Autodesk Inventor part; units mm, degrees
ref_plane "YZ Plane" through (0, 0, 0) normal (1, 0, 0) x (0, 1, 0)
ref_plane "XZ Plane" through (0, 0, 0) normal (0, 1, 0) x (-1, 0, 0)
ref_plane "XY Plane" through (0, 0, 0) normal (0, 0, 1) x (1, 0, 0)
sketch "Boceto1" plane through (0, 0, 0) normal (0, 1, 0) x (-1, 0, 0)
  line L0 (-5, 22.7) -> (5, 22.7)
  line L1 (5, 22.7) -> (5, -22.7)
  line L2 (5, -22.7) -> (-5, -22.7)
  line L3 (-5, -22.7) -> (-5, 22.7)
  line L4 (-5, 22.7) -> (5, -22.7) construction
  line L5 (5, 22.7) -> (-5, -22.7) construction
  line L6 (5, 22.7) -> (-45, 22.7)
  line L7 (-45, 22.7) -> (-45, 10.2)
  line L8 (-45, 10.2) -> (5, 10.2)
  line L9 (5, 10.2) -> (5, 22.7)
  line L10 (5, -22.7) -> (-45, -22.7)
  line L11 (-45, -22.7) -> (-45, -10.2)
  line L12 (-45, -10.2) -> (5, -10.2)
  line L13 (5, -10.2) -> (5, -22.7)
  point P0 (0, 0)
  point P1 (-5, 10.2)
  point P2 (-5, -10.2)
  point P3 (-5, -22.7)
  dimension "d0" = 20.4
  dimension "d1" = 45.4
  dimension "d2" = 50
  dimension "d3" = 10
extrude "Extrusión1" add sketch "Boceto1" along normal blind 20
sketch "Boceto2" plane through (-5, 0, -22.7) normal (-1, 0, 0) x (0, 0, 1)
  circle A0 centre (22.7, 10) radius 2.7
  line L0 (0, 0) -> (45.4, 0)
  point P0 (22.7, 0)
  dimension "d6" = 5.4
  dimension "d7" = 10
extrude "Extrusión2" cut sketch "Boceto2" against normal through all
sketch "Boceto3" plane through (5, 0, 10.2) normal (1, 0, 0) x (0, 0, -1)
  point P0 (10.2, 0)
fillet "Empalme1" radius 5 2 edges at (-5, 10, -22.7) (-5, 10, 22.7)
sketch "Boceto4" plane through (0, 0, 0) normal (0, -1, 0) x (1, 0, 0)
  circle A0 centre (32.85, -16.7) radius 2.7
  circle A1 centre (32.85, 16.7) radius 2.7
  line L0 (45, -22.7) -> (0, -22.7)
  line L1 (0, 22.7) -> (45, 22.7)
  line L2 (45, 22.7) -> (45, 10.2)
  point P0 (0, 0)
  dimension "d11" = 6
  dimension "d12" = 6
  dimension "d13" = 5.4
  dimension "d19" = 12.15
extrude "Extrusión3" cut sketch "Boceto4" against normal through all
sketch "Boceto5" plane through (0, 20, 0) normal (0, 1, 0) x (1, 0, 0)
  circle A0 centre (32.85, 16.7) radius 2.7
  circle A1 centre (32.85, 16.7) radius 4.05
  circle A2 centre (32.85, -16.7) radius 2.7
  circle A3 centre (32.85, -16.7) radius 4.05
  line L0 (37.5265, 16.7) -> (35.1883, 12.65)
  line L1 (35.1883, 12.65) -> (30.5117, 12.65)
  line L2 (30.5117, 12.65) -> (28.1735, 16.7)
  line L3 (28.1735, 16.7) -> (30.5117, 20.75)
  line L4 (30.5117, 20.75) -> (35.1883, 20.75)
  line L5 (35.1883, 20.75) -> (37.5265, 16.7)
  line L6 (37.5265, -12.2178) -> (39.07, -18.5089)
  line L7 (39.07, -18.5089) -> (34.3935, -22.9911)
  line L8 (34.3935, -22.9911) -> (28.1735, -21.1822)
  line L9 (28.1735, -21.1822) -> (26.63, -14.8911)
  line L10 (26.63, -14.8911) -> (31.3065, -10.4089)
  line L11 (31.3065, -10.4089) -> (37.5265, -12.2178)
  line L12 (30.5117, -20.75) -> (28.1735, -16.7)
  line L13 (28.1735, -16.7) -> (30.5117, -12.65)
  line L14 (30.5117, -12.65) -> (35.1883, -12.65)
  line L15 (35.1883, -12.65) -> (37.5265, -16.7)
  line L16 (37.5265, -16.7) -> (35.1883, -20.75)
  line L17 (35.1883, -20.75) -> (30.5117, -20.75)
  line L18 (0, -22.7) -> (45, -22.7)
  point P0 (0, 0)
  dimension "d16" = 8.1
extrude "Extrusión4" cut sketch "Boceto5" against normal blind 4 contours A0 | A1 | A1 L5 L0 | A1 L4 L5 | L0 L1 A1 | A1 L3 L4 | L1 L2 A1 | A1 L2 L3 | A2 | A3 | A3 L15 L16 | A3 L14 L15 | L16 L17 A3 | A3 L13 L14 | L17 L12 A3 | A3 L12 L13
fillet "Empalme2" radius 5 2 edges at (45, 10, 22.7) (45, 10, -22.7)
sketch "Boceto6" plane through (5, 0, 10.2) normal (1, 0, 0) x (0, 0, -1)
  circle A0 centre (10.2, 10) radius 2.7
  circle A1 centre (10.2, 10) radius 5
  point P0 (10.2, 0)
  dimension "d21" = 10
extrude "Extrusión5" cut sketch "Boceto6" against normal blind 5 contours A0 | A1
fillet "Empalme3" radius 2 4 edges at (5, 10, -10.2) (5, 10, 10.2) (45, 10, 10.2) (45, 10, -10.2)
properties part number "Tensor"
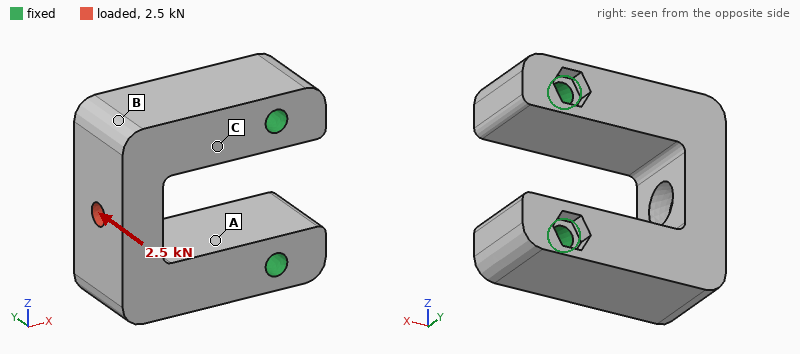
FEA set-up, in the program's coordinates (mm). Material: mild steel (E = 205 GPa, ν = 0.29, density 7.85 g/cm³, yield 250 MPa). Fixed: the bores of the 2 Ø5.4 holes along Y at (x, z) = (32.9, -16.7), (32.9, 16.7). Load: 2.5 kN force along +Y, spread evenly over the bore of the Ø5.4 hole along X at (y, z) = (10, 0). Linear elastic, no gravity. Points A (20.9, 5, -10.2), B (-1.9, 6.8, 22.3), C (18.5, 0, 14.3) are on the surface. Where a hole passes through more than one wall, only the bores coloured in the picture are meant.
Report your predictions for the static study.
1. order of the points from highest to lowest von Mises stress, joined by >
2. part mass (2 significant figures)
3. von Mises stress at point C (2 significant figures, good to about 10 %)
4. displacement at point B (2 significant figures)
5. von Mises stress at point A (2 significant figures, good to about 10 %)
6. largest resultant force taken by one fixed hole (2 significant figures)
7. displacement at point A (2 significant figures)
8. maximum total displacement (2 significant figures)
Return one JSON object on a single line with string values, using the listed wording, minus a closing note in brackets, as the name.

{"order of the points from highest to lowest von Mises stress, joined by >": "C > A > B", "part mass": "210 g", "von Mises stress at point C": "34 MPa", "displacement at point B": "15 µm", "von Mises stress at point A": "26 MPa", "largest resultant force taken by one fixed hole": "1.3 kN", "displacement at point A": "3.5 µm", "maximum total displacement": "21 µm"}
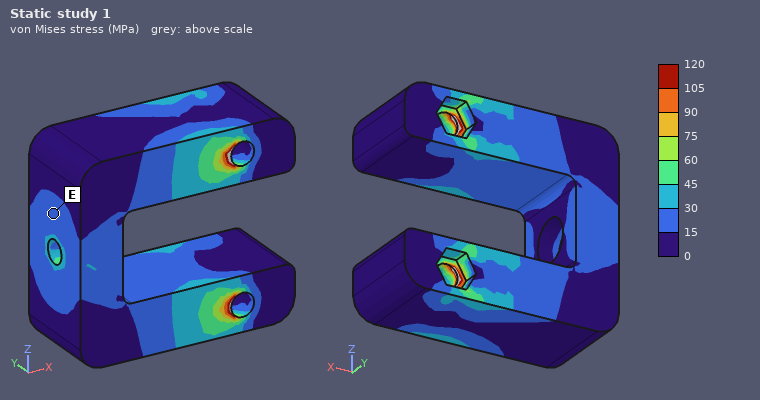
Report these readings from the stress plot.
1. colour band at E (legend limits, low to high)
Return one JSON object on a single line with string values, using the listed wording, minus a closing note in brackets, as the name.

{"colour band at E": "15 to 30 MPa"}
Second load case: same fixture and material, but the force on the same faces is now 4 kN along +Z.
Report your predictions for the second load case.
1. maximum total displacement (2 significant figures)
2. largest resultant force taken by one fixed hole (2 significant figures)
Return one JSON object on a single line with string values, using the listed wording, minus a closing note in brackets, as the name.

{"maximum total displacement": "21 µm", "largest resultant force taken by one fixed hole": "3.0 kN"}
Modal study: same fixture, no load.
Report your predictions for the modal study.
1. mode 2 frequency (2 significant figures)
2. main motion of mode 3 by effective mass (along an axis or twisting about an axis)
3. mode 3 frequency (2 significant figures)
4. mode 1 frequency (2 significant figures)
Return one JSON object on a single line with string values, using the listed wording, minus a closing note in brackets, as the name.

{"mode 2 frequency": "7500 Hz", "main motion of mode 3 by effective mass": "twisting about X", "mode 3 frequency": "11 kHz", "mode 1 frequency": "7300 Hz"}
